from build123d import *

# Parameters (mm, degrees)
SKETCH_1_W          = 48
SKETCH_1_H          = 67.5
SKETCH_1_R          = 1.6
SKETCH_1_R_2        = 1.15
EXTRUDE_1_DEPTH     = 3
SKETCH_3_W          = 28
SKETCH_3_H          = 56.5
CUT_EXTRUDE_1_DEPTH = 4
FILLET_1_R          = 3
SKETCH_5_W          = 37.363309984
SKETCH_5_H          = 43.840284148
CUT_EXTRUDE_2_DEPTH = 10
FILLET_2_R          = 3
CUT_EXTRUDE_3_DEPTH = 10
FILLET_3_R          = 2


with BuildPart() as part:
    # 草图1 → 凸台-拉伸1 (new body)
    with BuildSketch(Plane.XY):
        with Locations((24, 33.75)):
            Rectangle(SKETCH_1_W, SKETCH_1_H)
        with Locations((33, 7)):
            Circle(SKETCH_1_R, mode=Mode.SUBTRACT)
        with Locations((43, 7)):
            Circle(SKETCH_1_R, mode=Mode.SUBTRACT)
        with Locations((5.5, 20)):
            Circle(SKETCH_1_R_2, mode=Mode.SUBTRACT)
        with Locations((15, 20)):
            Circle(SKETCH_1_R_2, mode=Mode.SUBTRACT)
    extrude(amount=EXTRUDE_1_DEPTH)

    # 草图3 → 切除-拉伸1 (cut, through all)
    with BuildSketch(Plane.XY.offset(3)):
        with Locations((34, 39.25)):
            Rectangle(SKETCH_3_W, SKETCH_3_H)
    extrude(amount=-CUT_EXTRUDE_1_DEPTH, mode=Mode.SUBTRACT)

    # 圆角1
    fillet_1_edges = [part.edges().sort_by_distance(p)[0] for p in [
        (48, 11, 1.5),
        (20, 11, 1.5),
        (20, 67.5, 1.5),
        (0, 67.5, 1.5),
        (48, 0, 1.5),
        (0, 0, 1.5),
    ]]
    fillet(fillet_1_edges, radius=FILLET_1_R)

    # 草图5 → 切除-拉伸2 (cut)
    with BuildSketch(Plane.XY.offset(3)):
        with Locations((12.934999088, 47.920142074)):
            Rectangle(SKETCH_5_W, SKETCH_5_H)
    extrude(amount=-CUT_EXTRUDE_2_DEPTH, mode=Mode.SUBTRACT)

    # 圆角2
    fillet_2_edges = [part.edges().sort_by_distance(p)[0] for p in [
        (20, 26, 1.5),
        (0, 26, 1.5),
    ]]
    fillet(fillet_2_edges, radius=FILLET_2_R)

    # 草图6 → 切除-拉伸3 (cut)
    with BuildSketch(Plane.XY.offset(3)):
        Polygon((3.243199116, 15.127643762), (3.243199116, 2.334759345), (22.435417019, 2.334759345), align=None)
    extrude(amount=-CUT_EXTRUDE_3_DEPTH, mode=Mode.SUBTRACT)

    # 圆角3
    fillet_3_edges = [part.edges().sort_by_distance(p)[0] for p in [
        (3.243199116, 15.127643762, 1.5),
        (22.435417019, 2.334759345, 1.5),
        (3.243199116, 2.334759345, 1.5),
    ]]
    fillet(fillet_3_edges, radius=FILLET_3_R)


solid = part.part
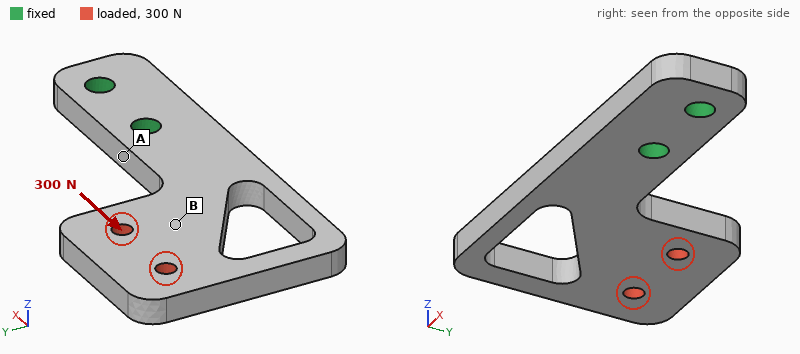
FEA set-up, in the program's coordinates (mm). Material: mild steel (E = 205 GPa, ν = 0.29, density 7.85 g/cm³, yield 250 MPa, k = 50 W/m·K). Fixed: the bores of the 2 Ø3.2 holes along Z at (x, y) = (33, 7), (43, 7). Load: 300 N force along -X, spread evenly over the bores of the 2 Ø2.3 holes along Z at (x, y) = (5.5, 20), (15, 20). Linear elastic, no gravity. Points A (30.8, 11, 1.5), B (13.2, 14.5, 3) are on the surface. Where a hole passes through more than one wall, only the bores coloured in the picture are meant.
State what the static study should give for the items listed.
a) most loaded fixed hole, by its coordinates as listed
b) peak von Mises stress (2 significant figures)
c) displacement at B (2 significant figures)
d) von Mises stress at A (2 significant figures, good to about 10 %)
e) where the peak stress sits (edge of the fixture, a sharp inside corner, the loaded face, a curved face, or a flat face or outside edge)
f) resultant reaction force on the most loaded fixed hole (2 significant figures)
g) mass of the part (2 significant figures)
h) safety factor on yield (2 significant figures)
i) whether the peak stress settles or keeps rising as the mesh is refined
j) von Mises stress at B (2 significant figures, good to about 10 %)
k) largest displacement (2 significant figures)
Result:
(33, 7)
190 MPa
24 µm
71 MPa
a curved face
470 N
16 g
1.3
settles
23 MPa
56 µm
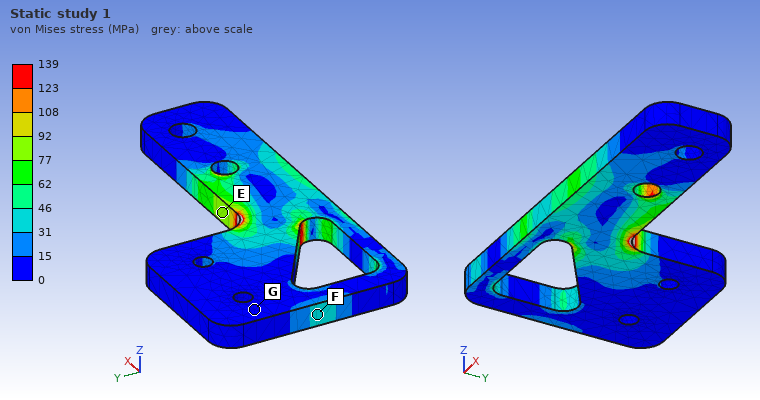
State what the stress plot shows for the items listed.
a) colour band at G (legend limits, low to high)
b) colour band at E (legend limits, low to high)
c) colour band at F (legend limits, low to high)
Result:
0 to 15 MPa
77 to 92 MPa
31 to 46 MPa
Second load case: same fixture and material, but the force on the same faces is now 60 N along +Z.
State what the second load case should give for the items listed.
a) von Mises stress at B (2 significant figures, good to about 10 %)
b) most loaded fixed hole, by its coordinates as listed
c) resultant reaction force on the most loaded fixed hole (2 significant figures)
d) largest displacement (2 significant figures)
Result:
19 MPa
(33, 7)
77 N
0.13 mm
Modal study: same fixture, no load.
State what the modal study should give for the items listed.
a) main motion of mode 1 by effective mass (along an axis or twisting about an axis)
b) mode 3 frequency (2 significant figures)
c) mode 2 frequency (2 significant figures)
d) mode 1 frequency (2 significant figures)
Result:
along Z
4000 Hz
3900 Hz
1600 Hz
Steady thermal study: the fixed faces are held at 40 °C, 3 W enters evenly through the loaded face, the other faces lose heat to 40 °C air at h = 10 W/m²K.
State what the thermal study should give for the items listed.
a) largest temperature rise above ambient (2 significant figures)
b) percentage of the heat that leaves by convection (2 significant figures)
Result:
46 K
15 %
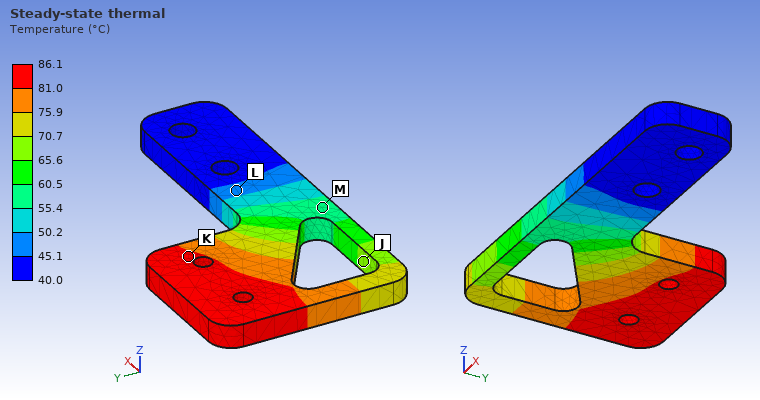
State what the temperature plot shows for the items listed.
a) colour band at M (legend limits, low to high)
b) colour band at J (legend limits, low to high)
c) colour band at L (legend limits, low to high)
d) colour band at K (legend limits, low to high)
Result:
55.4 to 60.5 °C
65.6 to 70.7 °C
45.1 to 50.2 °C
81.0 to 86.1 °C
